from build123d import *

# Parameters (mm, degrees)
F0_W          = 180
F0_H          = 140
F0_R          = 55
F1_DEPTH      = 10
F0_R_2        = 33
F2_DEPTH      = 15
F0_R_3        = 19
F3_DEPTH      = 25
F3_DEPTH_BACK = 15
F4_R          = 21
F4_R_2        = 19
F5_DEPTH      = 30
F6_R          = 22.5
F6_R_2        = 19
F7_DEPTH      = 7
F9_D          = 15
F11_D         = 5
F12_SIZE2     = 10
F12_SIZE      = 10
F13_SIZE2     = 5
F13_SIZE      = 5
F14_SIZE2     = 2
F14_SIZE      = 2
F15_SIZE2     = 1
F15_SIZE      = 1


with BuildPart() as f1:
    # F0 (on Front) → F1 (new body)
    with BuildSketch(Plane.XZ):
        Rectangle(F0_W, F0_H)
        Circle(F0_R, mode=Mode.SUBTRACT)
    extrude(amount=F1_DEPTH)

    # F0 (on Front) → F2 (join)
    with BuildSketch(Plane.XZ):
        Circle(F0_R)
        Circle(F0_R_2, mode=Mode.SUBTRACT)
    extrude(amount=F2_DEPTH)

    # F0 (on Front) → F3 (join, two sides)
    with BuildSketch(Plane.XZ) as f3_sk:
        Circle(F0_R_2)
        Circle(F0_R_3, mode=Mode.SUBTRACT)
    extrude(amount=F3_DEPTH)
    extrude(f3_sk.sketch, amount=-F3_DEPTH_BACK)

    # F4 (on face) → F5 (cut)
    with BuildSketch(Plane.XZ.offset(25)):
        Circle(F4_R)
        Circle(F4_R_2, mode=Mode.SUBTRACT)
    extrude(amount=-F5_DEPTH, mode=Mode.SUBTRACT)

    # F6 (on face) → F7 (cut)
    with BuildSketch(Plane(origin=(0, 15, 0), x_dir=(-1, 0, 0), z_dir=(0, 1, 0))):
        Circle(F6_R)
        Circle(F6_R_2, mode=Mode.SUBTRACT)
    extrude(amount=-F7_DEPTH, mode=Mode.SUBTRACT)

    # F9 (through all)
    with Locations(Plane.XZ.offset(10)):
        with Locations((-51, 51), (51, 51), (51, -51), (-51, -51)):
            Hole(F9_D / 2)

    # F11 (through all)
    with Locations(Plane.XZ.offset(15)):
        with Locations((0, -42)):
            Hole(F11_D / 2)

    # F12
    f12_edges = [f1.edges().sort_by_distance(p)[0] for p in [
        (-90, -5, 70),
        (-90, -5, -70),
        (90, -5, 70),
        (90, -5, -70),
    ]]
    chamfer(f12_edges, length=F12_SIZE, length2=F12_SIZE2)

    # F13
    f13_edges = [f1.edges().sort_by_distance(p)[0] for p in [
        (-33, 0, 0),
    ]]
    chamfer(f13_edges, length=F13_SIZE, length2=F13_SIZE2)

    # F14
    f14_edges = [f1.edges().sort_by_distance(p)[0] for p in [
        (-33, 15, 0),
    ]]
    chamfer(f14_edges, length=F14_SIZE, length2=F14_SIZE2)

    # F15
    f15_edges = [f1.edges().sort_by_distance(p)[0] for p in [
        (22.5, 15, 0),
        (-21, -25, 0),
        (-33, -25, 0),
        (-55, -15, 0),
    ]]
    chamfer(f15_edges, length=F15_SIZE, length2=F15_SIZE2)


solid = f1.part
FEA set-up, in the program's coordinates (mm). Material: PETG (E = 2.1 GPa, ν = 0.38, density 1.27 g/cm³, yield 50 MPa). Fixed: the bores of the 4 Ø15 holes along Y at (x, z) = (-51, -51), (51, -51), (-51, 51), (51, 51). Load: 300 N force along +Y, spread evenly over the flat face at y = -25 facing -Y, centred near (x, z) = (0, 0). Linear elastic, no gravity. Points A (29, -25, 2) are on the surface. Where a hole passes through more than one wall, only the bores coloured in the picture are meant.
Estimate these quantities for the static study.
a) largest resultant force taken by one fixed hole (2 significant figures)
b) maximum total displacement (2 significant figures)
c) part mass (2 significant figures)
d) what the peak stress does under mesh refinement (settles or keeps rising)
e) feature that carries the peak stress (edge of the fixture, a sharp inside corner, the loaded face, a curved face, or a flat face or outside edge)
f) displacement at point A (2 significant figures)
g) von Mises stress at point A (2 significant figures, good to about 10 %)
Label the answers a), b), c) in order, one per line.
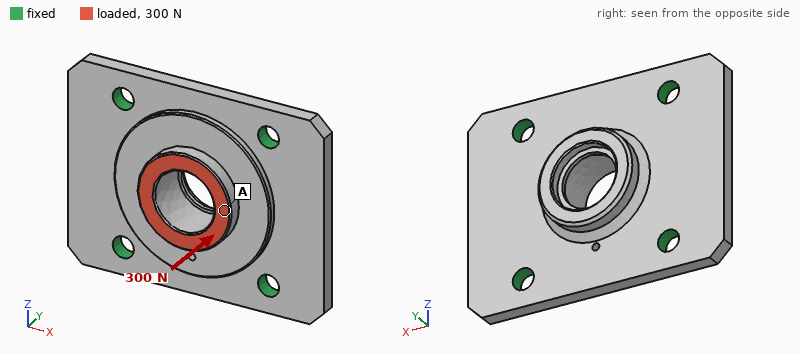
a) 83 N
b) 29 µm
c) 410 g
d) keeps rising
e) edge of the fixture
f) 28 µm
g) 0.25 MPa
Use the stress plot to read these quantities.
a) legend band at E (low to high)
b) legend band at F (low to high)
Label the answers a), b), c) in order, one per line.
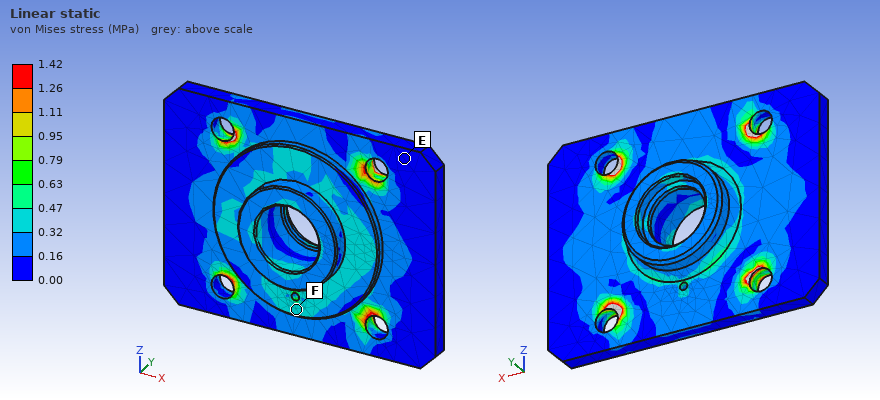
a) 0.00 to 0.16 MPa
b) 0.32 to 0.47 MPa
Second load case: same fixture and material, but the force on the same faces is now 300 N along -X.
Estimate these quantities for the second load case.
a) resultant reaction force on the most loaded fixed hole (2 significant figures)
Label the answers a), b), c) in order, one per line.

a) 86 N
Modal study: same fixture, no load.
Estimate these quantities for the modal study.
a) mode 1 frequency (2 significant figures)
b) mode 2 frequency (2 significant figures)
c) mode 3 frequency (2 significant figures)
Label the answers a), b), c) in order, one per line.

a) 1100 Hz
b) 1200 Hz
c) 1300 Hz
